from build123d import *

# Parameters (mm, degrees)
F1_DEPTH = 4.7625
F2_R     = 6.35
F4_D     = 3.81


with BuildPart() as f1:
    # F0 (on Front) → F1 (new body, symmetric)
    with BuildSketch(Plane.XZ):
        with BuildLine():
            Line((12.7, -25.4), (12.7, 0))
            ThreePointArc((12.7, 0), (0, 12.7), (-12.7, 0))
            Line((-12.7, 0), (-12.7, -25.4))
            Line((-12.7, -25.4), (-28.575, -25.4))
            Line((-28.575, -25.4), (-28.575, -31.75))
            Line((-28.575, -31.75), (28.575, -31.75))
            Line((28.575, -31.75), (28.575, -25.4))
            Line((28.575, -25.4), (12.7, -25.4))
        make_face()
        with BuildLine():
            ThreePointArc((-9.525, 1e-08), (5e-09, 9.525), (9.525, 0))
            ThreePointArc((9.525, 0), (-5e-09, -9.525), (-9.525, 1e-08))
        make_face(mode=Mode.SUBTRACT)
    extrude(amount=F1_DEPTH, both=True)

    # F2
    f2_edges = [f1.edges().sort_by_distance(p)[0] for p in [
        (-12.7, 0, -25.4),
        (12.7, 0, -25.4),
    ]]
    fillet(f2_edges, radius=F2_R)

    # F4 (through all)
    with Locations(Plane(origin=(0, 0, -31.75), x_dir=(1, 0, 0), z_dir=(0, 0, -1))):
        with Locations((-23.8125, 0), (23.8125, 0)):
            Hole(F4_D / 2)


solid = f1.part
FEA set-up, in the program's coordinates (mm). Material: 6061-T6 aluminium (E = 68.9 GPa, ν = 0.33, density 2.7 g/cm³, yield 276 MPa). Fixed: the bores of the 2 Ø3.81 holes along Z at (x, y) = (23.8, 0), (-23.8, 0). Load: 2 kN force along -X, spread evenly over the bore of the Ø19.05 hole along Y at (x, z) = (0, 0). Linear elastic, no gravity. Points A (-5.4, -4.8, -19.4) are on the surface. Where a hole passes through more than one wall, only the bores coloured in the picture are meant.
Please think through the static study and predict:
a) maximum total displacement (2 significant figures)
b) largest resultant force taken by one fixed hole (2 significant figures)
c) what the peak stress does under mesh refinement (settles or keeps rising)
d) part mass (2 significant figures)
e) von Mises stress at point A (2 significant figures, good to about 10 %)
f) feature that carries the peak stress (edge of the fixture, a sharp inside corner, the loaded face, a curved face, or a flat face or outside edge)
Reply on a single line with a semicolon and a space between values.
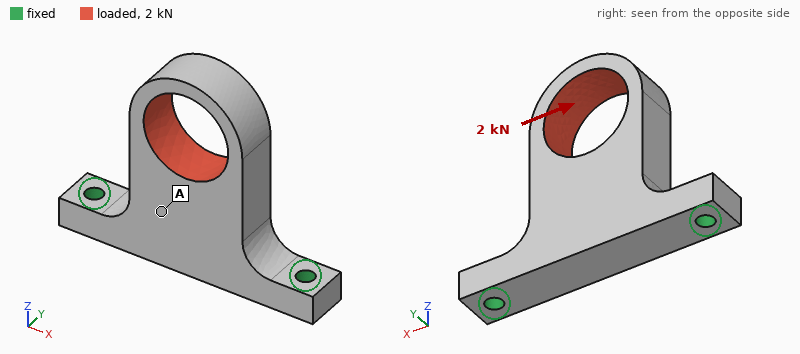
0.16 mm; 1.8 kN; keeps rising; 25 g; 18 MPa; edge of the fixture
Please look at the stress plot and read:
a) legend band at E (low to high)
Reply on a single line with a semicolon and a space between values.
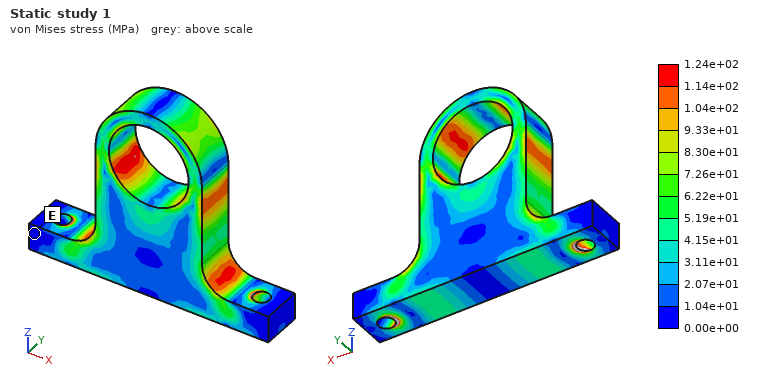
0.00e+00 to 1.04e+01 MPa
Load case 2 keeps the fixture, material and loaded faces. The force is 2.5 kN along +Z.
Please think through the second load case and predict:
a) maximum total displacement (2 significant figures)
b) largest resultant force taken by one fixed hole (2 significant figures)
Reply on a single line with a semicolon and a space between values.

45 µm; 1.4 kN
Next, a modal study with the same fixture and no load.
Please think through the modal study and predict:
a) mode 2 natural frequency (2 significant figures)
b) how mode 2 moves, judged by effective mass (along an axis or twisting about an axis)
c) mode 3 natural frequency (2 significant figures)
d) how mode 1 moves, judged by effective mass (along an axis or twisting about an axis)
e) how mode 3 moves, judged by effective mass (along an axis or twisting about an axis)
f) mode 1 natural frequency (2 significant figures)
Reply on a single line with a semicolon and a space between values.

8100 Hz; along X; 12 kHz; along Y; along Z; 2900 Hz
